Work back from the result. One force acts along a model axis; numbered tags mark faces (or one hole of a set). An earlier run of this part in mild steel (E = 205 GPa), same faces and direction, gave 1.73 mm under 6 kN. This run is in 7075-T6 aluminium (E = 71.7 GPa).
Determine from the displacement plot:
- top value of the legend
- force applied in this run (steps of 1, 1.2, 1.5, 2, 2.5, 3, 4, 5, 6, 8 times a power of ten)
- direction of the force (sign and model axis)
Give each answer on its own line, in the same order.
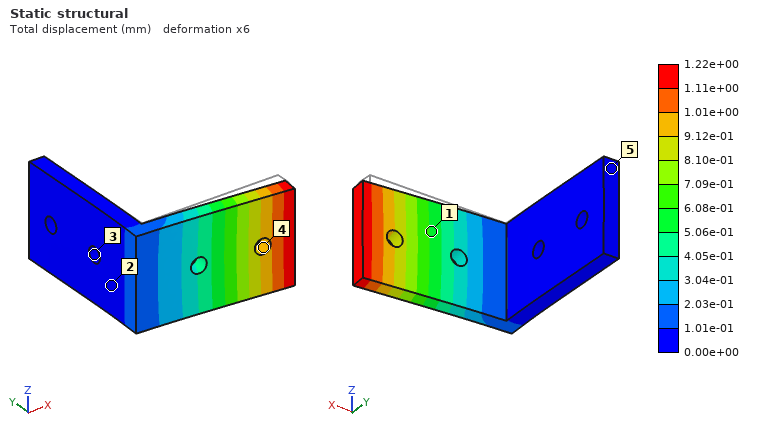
1.22e+00 mm
1.5 kN
-Y
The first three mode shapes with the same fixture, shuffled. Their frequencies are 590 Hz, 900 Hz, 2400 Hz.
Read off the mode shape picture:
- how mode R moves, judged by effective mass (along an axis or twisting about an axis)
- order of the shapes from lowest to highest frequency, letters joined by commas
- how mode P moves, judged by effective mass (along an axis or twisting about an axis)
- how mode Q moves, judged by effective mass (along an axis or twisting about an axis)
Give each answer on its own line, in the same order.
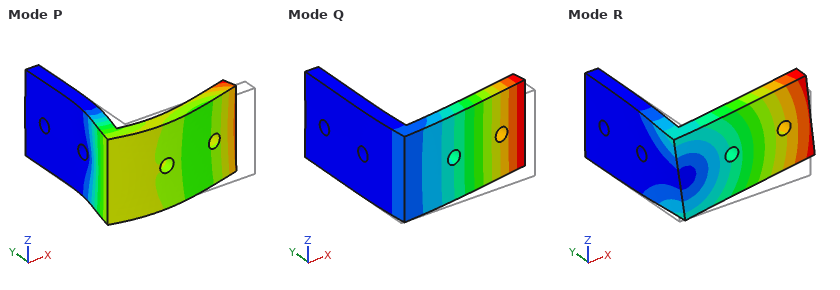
along Z
Q, R, P
along X
along Y
